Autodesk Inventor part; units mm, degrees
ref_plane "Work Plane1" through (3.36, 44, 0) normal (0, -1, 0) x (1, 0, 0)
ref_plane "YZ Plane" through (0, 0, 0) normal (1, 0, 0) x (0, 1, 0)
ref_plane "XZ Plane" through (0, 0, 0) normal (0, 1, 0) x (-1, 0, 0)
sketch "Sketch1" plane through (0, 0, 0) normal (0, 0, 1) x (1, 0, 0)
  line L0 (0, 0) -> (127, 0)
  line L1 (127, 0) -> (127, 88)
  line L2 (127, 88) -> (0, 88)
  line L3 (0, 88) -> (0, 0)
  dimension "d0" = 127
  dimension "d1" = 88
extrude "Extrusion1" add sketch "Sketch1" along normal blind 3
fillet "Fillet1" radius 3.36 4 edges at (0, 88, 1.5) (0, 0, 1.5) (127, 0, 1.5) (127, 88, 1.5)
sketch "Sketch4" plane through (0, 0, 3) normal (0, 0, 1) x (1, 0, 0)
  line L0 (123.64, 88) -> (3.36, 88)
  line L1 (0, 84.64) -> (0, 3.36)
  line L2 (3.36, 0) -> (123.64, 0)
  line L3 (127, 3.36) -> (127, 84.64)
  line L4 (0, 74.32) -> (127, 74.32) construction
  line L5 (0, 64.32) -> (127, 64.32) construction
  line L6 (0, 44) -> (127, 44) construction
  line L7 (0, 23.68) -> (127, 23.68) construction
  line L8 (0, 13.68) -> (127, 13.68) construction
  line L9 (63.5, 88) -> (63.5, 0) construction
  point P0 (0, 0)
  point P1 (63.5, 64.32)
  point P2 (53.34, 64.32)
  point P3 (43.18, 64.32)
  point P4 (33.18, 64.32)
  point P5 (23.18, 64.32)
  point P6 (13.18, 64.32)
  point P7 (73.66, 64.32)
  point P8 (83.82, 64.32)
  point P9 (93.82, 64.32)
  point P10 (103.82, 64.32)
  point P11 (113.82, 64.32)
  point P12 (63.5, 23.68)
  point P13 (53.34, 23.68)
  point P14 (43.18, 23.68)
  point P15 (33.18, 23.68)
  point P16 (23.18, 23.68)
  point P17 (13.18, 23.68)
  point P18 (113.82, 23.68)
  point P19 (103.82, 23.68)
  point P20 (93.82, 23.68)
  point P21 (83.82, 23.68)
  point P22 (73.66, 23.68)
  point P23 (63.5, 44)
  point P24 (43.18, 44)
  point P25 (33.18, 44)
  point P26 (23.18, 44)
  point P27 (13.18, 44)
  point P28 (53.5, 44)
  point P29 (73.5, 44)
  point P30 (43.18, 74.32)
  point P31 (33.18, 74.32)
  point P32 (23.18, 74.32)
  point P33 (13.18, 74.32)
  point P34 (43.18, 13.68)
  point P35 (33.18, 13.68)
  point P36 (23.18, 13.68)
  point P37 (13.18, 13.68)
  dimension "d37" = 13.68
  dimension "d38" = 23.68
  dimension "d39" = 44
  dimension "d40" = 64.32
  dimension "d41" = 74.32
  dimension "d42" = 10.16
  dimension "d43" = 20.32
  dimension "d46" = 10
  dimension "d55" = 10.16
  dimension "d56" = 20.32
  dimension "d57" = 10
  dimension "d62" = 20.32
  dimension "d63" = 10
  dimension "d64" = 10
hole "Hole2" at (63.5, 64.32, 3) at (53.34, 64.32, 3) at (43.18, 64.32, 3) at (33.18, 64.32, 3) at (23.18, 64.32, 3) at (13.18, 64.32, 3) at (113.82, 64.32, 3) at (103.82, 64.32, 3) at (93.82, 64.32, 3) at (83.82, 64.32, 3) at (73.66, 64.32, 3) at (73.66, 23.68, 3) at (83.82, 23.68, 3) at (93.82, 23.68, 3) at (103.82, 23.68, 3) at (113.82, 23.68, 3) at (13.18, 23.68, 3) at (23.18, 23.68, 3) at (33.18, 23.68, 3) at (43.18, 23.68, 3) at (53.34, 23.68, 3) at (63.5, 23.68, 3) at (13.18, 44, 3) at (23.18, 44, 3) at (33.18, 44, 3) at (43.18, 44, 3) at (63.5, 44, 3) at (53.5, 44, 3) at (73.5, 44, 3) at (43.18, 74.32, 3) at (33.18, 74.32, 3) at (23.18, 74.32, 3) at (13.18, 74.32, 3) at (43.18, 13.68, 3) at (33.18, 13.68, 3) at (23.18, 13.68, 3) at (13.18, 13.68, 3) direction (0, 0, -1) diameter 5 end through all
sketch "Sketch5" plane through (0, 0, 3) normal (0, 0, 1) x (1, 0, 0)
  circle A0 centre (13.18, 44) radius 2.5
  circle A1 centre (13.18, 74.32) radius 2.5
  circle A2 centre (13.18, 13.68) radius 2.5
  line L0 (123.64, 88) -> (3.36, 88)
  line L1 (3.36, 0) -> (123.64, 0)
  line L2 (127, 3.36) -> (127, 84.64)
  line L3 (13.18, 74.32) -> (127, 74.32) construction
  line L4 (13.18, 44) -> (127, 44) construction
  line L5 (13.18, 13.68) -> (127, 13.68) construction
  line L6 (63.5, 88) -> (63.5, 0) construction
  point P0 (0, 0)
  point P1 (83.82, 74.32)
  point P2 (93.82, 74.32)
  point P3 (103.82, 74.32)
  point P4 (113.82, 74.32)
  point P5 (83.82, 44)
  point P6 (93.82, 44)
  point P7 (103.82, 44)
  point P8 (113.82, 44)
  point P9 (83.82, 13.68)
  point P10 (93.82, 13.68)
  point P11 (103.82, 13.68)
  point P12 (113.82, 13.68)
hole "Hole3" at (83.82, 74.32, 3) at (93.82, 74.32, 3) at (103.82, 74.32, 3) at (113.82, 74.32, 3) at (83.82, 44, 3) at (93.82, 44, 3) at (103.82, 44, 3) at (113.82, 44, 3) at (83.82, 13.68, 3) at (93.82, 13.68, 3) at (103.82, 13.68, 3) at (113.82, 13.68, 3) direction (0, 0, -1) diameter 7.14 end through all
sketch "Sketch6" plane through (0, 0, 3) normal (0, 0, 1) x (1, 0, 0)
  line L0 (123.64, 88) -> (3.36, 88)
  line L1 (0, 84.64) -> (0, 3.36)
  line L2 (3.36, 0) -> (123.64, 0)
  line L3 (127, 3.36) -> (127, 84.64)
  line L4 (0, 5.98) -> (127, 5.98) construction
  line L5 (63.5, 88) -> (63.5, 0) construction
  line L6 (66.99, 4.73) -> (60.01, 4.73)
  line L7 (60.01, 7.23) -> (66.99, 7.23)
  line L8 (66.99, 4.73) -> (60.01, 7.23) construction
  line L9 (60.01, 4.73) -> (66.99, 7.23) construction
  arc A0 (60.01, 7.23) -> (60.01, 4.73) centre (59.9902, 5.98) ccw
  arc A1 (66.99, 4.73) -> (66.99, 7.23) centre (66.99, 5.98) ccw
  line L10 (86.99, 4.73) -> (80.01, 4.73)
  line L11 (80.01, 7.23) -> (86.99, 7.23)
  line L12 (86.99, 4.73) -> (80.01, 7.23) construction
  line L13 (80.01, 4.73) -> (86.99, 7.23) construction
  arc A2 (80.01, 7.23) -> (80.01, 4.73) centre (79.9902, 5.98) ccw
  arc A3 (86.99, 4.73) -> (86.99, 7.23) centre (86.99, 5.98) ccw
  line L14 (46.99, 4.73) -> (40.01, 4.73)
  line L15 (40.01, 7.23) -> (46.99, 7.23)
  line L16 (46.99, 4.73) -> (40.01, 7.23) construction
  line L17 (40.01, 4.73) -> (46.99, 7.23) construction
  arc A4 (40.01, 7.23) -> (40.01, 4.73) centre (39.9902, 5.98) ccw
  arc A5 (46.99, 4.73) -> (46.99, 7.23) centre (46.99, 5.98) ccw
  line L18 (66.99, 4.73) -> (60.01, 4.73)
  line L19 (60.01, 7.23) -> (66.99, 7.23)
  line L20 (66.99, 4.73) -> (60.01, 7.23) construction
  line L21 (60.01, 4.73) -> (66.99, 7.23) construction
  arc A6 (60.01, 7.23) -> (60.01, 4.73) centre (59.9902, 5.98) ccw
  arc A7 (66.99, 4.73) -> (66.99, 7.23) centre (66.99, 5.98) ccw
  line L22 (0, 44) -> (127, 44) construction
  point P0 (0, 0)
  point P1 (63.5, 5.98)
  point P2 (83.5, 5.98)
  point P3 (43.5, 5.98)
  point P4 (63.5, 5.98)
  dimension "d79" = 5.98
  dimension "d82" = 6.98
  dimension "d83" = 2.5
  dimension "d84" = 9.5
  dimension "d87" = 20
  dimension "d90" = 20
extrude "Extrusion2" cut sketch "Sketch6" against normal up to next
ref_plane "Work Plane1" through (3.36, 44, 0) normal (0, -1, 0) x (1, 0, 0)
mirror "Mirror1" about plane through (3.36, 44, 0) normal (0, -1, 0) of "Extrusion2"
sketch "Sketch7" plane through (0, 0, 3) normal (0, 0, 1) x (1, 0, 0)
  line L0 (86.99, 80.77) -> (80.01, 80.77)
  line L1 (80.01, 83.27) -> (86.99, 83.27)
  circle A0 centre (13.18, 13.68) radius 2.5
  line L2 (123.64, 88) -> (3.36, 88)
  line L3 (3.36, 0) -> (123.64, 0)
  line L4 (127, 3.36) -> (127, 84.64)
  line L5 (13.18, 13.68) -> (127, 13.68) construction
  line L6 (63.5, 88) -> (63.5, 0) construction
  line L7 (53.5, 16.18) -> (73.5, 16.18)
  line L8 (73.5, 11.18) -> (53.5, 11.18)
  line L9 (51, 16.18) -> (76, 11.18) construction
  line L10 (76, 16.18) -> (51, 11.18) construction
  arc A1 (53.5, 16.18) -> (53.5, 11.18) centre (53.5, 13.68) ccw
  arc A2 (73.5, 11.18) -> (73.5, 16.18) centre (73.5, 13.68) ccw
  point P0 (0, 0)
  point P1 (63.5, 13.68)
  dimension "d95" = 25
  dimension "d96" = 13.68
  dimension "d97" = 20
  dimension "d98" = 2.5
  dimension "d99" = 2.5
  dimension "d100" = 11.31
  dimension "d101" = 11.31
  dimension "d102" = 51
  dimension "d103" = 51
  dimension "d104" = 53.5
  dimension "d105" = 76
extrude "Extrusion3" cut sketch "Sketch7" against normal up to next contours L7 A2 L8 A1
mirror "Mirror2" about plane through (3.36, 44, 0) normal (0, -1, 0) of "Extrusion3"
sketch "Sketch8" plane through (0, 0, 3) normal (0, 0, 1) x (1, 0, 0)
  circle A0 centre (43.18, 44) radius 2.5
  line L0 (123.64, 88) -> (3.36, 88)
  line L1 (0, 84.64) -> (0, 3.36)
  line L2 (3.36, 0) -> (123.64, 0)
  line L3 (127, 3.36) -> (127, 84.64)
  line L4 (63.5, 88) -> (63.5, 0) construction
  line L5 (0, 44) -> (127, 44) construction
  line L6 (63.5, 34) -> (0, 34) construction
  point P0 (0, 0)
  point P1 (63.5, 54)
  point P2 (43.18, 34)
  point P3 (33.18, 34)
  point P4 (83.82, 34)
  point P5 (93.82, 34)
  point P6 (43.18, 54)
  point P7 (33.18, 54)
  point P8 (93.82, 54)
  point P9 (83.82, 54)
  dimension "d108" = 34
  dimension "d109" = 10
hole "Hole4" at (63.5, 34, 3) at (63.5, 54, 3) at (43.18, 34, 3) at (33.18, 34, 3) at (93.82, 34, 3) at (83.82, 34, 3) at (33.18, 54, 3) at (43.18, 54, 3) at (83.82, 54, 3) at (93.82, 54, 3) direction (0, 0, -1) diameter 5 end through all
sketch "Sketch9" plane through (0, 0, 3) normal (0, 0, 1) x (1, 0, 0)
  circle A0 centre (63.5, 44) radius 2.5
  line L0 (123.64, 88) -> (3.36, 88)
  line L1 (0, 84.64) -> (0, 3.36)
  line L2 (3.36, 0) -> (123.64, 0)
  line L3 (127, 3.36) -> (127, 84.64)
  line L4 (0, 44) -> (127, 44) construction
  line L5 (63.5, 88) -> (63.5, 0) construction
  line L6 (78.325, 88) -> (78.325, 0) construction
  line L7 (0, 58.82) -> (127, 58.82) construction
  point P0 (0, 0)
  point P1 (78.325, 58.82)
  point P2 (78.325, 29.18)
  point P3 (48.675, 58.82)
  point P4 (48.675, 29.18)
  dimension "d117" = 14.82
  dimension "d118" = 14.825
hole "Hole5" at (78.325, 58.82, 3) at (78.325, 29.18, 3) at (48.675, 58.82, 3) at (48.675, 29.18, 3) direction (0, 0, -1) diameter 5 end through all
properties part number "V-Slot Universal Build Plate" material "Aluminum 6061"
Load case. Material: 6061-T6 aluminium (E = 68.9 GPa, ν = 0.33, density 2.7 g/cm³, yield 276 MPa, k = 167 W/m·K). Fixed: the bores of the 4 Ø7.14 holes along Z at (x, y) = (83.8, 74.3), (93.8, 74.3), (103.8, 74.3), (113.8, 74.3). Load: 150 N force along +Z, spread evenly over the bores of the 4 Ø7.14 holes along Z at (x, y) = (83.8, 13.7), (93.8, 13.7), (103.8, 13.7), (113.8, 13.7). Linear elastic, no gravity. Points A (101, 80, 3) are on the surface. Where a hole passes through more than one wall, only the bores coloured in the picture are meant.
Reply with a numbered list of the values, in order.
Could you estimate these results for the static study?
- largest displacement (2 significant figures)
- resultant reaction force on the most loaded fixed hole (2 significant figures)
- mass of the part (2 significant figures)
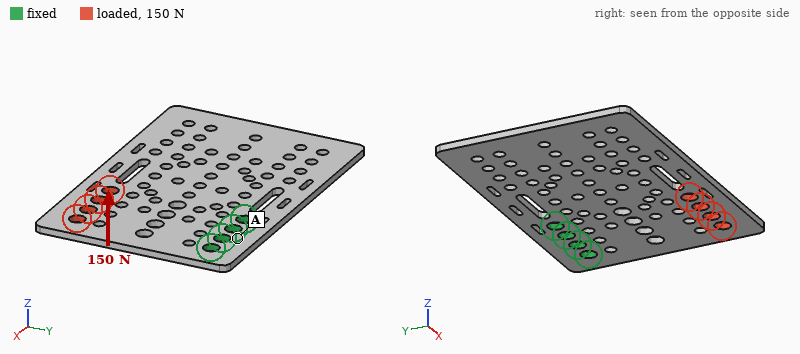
1. 1.6 mm
2. 45 N
3. 75 g
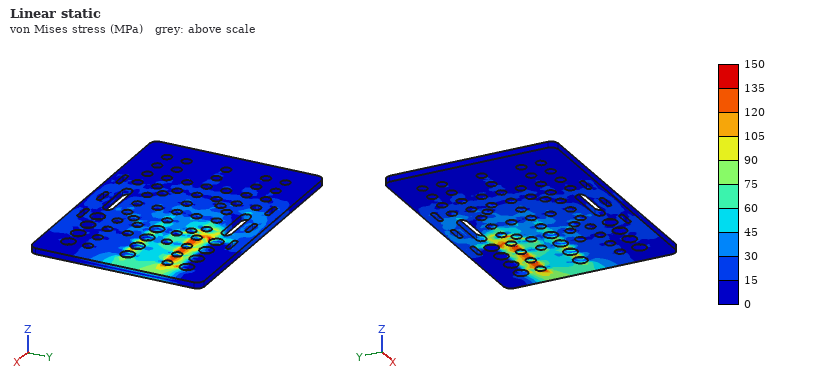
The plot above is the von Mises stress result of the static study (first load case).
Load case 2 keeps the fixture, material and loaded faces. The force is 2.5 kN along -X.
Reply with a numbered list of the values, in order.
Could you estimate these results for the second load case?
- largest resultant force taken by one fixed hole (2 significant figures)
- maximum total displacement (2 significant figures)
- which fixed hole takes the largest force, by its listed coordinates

1. 4.1 kN
2. 0.31 mm
3. (113.8, 74.3)
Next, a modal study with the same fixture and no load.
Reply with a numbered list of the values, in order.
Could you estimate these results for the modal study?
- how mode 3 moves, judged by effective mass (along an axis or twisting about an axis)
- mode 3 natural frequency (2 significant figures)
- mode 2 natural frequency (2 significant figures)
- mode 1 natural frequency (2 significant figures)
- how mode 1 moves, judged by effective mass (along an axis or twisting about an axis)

1. along Z
2. 760 Hz
3. 410 Hz
4. 220 Hz
5. along Z
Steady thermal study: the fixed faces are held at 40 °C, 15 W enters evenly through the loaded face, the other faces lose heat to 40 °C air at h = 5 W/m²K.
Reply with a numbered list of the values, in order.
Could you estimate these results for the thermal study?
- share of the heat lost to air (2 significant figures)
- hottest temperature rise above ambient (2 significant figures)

1. 11 %
2. 37 K
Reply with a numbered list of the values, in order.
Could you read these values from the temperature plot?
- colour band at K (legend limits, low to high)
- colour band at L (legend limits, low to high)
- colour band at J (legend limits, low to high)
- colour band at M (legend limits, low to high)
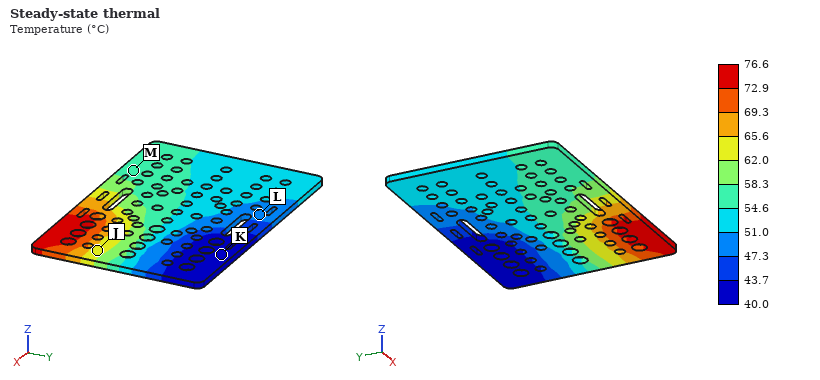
1. 40.0 to 43.7 °C
2. 47.3 to 51.0 °C
3. 62.0 to 65.6 °C
4. 54.6 to 58.3 °C
